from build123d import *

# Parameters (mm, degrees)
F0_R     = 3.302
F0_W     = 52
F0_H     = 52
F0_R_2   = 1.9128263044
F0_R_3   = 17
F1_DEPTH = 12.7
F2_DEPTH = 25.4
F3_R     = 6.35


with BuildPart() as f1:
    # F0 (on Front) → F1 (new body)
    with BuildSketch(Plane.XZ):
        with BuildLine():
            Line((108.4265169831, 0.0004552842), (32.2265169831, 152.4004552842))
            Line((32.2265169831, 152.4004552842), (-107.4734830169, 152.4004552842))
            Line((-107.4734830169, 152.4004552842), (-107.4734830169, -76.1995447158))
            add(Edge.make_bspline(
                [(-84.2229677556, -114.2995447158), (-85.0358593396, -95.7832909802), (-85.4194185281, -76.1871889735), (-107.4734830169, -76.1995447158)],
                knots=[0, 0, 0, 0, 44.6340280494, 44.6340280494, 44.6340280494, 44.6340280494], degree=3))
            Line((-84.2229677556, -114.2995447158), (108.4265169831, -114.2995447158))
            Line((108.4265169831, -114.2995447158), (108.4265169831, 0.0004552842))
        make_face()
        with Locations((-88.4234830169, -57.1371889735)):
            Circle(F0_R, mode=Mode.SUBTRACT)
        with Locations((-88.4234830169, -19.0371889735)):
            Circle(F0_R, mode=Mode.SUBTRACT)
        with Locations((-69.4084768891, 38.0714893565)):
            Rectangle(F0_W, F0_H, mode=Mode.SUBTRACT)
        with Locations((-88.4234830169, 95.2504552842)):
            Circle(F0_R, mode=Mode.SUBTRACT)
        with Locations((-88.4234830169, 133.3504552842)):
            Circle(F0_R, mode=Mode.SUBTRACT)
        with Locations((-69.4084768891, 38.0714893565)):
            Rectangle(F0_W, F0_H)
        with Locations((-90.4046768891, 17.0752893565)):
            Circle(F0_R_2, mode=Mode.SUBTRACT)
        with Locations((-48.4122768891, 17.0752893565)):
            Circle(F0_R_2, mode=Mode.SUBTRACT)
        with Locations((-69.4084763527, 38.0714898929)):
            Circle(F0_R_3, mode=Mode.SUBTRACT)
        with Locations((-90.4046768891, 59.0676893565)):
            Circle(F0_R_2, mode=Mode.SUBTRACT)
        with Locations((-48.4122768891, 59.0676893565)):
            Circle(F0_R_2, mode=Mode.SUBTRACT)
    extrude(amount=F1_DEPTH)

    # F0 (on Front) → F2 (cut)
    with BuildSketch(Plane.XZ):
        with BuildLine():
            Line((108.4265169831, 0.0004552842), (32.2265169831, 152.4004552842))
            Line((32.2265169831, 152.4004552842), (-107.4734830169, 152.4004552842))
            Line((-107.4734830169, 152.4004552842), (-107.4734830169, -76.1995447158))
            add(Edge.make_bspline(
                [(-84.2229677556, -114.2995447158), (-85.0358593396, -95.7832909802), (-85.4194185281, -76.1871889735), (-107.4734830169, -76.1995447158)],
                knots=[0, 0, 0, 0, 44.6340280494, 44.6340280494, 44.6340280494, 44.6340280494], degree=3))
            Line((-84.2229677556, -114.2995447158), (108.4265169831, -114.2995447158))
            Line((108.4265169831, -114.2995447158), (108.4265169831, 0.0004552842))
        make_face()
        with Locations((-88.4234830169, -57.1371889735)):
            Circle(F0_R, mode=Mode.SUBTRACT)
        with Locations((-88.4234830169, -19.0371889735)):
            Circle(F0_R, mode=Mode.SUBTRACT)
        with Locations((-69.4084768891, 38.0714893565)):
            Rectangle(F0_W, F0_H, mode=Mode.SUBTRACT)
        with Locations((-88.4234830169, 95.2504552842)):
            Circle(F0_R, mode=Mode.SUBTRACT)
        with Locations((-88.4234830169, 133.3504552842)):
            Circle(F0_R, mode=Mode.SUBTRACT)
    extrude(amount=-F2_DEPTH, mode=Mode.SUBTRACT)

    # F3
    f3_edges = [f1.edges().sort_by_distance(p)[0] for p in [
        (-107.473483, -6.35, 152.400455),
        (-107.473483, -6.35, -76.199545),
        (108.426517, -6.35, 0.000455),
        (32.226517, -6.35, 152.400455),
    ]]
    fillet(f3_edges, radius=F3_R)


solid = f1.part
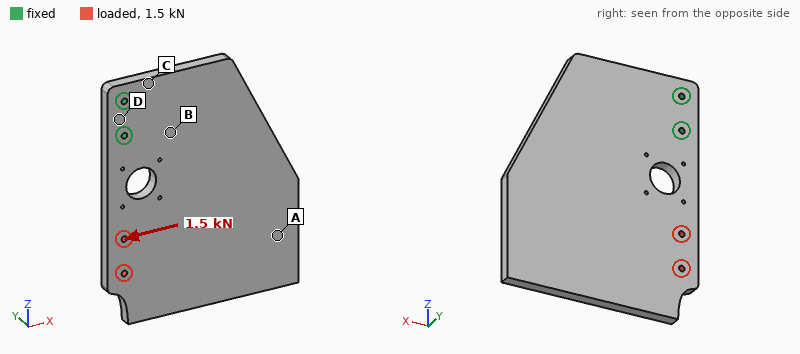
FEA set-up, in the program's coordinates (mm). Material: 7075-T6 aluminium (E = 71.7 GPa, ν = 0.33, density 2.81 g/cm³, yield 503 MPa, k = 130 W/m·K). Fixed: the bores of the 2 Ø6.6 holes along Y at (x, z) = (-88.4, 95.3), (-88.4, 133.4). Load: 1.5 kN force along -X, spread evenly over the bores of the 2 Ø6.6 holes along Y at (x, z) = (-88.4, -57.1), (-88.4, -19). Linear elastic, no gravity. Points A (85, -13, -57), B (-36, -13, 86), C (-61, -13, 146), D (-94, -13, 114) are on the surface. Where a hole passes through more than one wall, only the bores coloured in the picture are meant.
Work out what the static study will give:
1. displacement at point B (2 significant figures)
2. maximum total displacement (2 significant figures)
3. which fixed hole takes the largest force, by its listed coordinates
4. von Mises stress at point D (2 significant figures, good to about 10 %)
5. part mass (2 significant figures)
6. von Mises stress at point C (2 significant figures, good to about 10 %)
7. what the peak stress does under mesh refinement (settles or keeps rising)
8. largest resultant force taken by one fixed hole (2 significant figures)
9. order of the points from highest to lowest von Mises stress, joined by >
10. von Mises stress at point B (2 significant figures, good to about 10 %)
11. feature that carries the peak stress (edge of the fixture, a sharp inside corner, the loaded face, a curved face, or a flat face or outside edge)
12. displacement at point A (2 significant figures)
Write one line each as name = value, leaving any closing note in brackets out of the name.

displacement at point B = 0.020 mm
maximum total displacement = 0.12 mm
which fixed hole takes the largest force, by its listed coordinates = (-88.4, 95.3)
von Mises stress at point D = 5.6 MPa
part mass = 1.8 kg
von Mises stress at point C = 7.9 MPa
what the peak stress does under mesh refinement = keeps rising
largest resultant force taken by one fixed hole = 6.2 kN
order of the points from highest to lowest von Mises stress, joined by > = C > D > B > A
von Mises stress at point B = 4.0 MPa
feature that carries the peak stress = edge of the fixture
displacement at point A = 0.099 mm
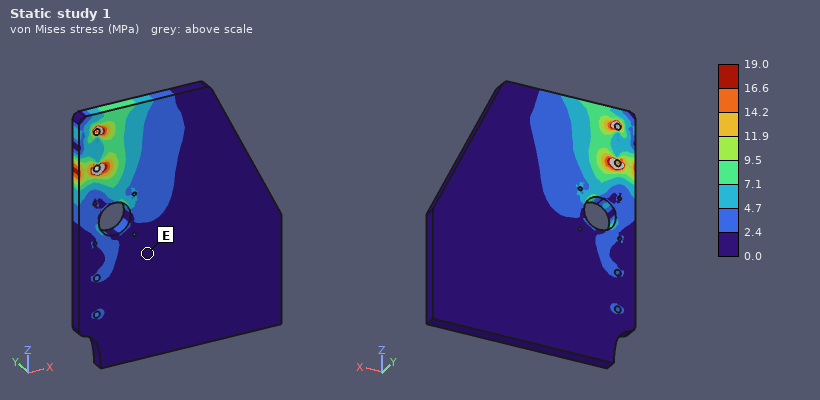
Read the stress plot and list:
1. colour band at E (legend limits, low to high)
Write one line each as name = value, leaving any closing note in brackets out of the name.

colour band at E = 0.0 to 2.4 MPa
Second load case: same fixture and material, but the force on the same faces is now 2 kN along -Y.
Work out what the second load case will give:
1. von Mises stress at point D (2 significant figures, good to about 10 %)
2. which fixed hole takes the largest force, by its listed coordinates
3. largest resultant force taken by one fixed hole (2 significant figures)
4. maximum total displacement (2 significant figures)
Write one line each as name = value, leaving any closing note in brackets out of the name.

von Mises stress at point D = 21 MPa
which fixed hole takes the largest force, by its listed coordinates = (-88.4, 95.3)
largest resultant force taken by one fixed hole = 5.8 kN
maximum total displacement = 2.7 mm
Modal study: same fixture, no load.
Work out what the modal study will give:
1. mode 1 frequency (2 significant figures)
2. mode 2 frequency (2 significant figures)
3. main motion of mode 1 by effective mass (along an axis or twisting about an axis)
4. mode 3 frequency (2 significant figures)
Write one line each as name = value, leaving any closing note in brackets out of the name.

mode 1 frequency = 130 Hz
mode 2 frequency = 300 Hz
main motion of mode 1 by effective mass = along Y
mode 3 frequency = 560 Hz
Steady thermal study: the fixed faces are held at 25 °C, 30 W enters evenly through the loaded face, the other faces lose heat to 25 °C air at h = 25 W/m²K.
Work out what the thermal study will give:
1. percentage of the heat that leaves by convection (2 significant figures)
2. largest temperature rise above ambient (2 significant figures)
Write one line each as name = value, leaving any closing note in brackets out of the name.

percentage of the heat that leaves by convection = 62 %
largest temperature rise above ambient = 18 K
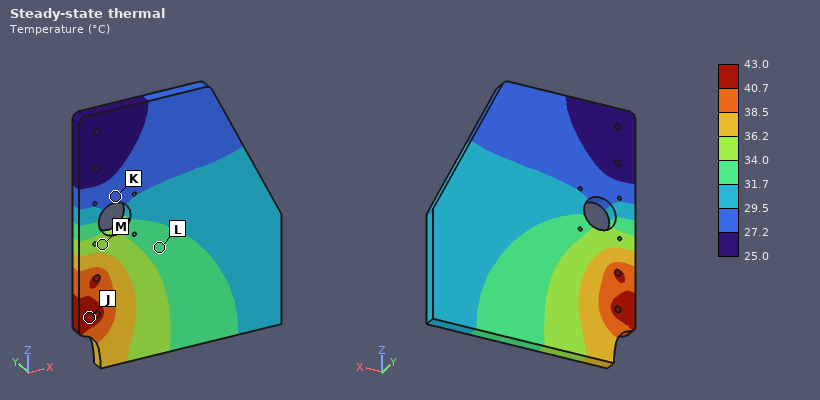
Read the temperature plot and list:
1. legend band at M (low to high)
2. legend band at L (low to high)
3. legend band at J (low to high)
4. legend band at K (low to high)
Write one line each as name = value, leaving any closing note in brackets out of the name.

legend band at M = 34.0 to 36.2 °C
legend band at L = 31.7 to 34.0 °C
legend band at J = 40.7 to 43.0 °C
legend band at K = 27.2 to 29.5 °C
